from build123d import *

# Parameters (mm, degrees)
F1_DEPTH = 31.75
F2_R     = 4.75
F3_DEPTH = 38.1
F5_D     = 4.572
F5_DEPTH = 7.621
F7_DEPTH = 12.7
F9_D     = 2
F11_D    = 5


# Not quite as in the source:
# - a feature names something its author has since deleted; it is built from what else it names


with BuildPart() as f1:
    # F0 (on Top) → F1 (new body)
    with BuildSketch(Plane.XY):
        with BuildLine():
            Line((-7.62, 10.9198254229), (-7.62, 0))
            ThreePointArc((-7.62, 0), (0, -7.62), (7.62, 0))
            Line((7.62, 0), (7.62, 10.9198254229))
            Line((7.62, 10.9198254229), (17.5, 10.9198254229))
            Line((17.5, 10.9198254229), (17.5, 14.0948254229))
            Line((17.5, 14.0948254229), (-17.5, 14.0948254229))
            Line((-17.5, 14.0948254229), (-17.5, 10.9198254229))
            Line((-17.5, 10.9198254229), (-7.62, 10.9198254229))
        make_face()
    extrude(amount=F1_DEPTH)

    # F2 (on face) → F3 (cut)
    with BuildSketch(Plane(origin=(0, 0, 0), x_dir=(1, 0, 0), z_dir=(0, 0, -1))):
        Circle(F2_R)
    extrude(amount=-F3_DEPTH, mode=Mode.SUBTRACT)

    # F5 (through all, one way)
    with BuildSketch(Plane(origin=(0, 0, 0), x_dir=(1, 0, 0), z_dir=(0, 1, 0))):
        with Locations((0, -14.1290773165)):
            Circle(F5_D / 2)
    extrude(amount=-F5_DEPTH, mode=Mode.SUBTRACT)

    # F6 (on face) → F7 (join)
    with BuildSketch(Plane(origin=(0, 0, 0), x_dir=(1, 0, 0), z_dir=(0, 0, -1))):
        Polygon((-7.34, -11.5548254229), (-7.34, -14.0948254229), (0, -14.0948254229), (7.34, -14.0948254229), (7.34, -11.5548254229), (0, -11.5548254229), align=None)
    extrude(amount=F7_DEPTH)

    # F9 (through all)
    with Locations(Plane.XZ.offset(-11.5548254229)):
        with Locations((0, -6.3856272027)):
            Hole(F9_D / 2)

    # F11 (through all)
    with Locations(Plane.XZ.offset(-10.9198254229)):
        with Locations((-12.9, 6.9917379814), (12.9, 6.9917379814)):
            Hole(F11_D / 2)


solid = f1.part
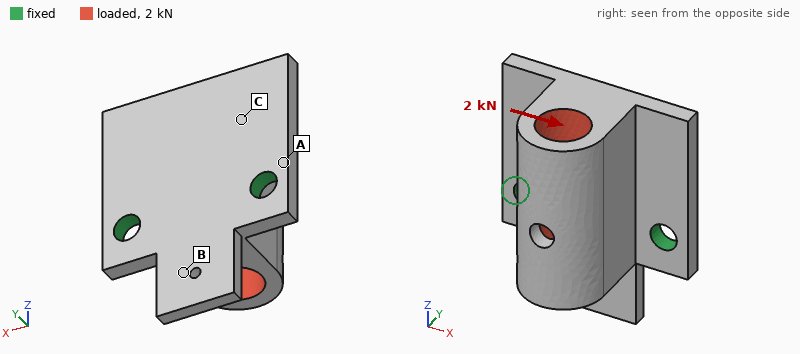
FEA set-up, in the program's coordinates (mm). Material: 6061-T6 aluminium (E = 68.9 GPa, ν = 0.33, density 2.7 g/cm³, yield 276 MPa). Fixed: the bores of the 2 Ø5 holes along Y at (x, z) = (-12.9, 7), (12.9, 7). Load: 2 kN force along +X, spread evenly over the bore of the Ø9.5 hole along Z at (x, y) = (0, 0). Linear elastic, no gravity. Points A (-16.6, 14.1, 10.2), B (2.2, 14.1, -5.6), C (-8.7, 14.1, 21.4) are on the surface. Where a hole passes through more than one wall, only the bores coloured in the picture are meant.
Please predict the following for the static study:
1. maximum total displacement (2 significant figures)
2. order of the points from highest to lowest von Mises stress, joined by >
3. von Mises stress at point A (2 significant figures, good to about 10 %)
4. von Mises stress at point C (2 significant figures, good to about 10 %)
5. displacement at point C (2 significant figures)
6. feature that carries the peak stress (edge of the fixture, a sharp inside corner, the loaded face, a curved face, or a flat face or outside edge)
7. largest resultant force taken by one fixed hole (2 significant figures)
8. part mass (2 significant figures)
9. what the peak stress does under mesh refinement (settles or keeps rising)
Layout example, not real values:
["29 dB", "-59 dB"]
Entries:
["52 µm", "A > C > B", "50 MPa", "23 MPa", "16 µm", "edge of the fixture", "1.7 kN", "26 g", "keeps rising"]
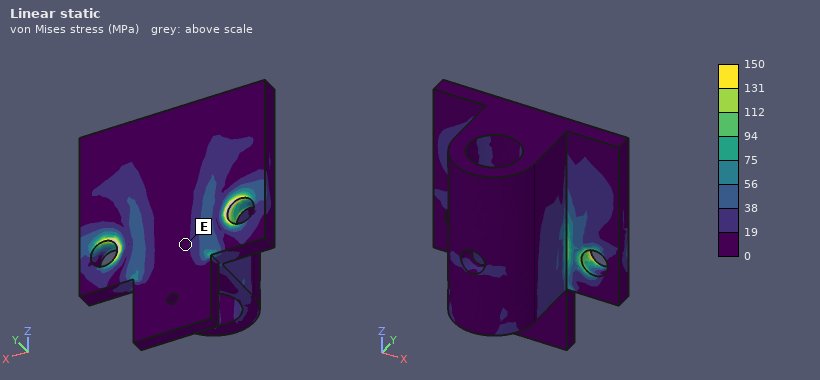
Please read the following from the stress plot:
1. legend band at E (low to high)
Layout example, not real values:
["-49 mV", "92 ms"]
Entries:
["0 to 19 MPa"]
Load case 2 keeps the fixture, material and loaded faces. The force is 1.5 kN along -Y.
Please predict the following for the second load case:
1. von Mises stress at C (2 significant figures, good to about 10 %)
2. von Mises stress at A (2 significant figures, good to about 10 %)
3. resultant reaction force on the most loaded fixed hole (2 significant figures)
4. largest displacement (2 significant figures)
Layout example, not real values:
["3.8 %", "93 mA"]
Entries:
["35 MPa", "95 MPa", "800 N", "0.16 mm"]
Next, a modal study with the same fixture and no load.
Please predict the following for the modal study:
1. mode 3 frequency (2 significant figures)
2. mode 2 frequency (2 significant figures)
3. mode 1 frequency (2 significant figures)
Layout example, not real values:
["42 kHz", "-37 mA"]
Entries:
["10 kHz", "10 kHz", "3400 Hz"]
